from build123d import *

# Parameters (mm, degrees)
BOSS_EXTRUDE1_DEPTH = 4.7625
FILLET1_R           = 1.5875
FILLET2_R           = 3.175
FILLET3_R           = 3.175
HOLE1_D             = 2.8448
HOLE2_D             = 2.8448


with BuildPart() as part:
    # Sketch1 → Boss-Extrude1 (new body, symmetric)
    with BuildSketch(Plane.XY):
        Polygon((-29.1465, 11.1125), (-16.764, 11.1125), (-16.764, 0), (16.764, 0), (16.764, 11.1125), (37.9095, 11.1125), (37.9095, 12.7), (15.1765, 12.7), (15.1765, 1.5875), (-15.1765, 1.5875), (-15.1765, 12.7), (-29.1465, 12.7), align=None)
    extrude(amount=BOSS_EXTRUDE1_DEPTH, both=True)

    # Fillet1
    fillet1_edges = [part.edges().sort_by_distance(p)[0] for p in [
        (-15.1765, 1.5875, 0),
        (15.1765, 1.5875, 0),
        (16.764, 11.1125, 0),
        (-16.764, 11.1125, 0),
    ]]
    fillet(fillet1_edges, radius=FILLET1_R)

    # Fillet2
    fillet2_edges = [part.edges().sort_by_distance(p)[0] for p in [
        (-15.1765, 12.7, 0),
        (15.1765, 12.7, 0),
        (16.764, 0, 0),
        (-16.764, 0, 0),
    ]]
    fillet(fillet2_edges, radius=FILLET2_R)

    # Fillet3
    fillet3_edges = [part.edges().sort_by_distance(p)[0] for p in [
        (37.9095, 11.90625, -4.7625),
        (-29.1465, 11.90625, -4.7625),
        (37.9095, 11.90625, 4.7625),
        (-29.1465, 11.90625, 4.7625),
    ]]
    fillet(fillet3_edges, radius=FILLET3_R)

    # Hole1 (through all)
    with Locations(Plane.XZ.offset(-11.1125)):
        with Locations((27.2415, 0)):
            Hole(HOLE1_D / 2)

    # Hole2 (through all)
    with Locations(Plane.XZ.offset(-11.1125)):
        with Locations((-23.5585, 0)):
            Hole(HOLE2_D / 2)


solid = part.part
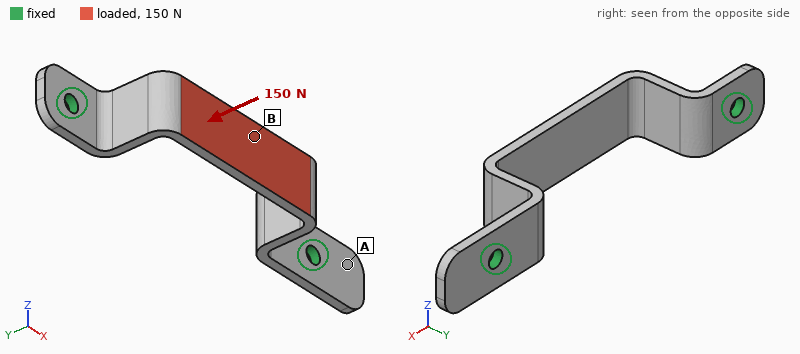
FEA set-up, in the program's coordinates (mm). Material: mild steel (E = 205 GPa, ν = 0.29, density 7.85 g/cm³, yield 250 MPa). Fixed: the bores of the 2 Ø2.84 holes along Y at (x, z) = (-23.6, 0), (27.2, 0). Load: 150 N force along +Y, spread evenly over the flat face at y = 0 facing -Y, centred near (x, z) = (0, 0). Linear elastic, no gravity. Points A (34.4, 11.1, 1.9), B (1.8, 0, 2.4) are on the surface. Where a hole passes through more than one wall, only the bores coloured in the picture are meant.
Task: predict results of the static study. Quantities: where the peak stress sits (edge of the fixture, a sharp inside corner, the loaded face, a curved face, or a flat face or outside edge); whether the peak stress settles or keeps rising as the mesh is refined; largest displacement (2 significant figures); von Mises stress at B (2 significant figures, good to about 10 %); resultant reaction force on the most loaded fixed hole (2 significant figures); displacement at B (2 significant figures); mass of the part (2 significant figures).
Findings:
edge of the fixture
keeps rising
38 µm
67 MPa
100 N
37 µm
9.8 g
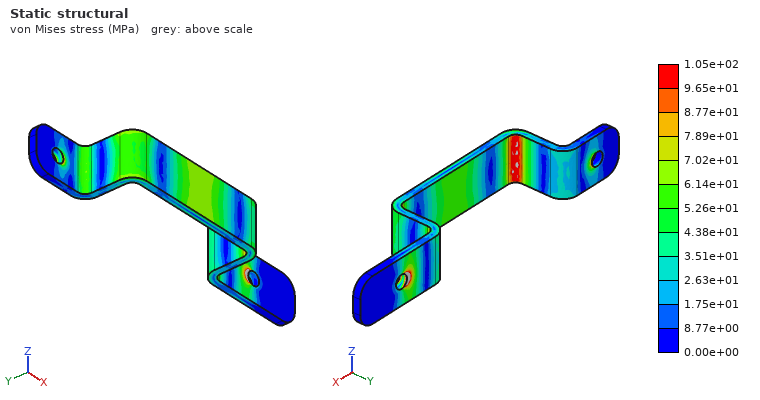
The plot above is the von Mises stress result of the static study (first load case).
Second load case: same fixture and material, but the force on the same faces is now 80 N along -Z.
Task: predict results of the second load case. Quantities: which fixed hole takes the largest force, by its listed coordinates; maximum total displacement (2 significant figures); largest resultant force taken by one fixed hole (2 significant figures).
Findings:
(-23.6, 0)
50 µm
43 N
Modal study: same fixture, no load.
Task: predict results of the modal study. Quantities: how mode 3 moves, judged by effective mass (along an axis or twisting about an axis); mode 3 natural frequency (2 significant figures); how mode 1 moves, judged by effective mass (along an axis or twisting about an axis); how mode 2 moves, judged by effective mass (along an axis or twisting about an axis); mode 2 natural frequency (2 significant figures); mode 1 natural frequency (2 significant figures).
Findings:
along Y
5900 Hz
along Z
along X
4200 Hz
3400 Hz
